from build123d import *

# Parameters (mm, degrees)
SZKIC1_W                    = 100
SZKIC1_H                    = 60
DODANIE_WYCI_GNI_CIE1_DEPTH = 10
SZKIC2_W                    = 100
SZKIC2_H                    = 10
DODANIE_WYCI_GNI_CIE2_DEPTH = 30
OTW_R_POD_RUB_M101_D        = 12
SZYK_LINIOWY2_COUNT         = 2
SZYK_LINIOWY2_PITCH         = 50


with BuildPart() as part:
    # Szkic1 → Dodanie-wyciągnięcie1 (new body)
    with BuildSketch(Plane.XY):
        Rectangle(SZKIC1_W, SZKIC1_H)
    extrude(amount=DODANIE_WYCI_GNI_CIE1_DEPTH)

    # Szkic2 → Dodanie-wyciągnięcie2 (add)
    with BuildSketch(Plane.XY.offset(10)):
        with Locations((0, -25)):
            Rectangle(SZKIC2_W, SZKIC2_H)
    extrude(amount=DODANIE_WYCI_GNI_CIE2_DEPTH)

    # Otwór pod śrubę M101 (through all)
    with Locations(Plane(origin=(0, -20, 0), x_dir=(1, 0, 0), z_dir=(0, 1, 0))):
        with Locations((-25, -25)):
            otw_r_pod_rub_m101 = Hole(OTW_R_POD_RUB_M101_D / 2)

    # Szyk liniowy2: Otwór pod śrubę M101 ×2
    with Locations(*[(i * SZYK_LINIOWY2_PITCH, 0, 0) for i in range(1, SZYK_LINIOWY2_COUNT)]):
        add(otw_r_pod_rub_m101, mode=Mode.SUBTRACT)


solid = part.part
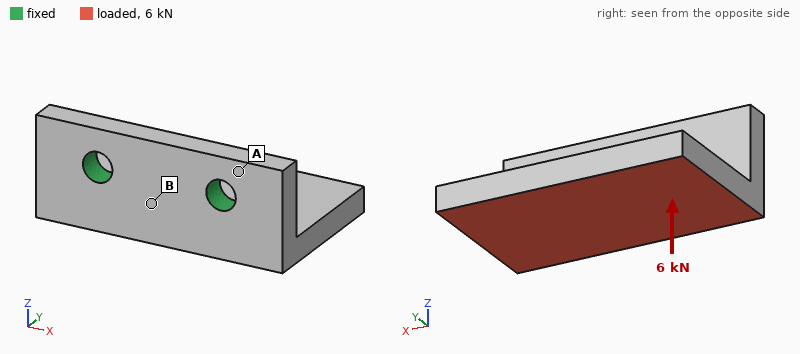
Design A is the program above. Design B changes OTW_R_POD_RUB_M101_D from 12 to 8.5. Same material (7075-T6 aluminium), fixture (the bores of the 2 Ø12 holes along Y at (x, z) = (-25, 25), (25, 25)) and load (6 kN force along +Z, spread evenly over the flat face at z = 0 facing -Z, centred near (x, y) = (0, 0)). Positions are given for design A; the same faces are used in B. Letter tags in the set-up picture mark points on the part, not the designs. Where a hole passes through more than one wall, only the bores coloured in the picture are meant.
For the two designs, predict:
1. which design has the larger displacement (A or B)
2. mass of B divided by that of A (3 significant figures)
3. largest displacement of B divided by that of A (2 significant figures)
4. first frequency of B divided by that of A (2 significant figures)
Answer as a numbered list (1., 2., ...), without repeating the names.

1. B
2. 1.01
3. 1.1
4. 0.94
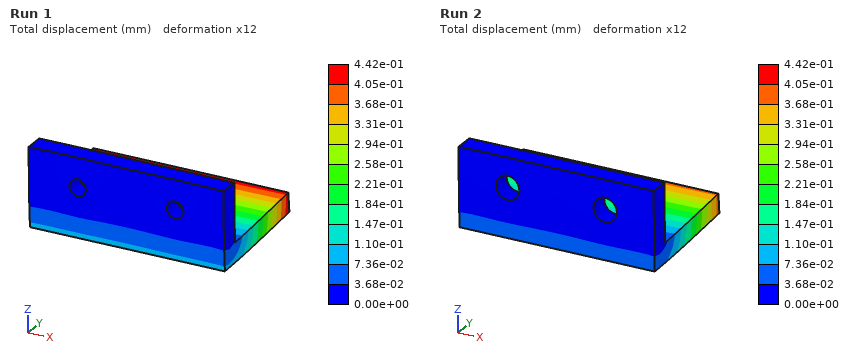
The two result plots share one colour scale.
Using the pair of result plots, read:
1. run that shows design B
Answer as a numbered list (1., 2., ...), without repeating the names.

1. Run 1
